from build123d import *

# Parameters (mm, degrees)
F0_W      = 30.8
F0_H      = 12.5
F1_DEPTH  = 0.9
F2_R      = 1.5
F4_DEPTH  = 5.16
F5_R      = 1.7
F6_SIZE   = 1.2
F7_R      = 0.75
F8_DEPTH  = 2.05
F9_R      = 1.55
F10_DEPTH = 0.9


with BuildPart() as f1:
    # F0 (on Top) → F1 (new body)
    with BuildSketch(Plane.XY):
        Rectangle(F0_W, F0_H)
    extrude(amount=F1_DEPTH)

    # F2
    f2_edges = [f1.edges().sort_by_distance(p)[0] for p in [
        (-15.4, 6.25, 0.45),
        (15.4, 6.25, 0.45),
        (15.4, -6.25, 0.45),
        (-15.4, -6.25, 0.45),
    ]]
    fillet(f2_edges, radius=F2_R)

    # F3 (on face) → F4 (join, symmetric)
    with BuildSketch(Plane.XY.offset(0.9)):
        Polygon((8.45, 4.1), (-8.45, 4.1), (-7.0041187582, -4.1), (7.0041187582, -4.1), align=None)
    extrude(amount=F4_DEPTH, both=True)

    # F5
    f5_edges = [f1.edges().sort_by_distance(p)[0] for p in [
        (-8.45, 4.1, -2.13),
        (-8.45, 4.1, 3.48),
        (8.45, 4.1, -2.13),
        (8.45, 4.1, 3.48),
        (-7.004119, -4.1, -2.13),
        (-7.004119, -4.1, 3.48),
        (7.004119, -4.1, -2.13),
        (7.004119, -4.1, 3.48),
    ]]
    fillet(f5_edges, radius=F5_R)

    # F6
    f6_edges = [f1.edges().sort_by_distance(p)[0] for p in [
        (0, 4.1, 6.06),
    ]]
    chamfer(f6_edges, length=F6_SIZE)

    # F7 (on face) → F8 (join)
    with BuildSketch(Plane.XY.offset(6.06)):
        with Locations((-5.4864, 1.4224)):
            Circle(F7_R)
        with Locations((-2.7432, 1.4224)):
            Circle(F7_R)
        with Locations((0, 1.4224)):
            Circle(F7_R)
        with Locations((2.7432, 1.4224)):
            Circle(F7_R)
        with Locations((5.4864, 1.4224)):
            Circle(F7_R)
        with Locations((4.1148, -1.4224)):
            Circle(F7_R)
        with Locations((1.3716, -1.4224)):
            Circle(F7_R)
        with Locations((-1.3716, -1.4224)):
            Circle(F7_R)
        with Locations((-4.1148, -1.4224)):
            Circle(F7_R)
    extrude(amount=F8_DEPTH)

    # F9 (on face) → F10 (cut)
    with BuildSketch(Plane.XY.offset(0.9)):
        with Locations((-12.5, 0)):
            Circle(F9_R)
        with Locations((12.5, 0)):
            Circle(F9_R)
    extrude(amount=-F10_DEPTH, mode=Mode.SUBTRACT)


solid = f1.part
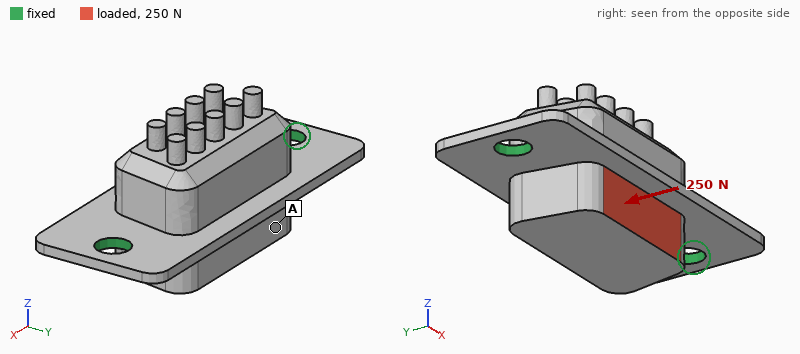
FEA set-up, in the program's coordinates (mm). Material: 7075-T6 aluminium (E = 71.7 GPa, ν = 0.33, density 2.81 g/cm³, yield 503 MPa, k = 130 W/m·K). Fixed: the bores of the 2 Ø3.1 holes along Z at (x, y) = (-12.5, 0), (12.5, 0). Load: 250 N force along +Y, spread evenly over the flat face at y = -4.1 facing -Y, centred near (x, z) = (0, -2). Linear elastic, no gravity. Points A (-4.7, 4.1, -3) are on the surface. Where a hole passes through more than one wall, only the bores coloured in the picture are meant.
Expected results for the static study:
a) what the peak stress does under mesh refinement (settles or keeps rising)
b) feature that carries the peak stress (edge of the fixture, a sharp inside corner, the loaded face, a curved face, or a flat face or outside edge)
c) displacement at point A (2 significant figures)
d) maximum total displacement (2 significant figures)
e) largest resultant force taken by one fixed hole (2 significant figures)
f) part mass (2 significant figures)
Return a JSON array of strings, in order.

["keeps rising", "edge of the fixture", "53 µm", "73 µm", "130 N", "4.2 g"]
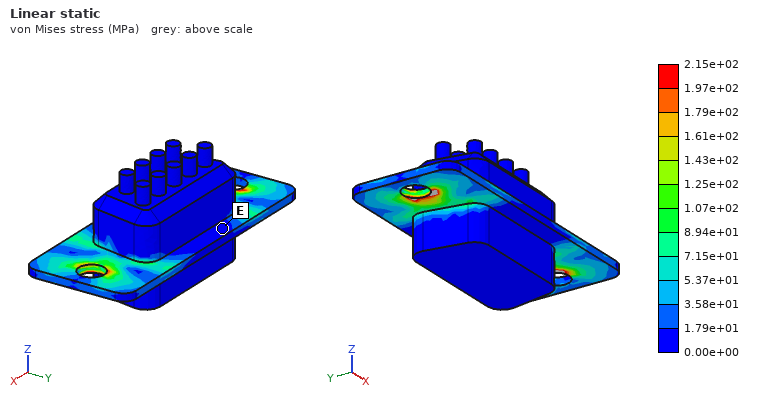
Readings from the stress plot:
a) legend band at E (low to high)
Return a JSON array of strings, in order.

["0.00e+00 to 1.79e+01 MPa"]
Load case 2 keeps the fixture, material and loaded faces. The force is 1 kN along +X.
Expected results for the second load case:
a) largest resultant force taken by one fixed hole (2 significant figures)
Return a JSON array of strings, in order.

["550 N"]
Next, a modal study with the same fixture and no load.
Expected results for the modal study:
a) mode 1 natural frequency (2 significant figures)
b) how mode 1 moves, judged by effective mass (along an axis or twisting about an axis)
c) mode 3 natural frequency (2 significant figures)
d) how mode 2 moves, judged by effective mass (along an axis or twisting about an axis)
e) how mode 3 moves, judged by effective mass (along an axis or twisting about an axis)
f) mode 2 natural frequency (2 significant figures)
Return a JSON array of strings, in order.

["5300 Hz", "twisting about X", "16 kHz", "along Z", "twisting about Y", "8900 Hz"]
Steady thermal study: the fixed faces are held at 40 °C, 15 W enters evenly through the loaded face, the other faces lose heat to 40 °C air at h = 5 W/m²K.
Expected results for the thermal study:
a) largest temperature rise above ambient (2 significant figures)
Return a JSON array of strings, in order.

["40 K"]
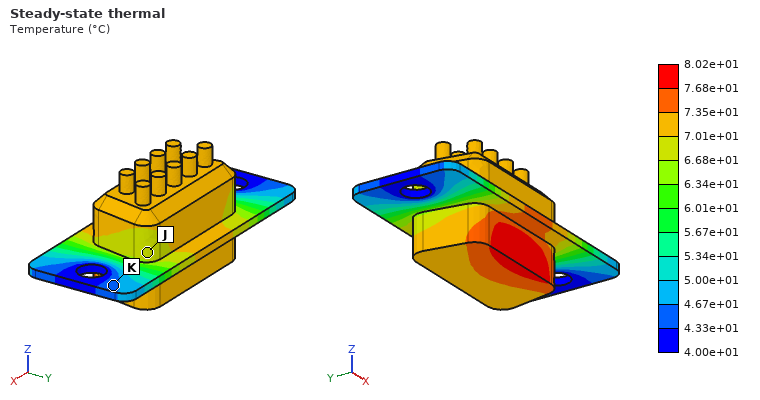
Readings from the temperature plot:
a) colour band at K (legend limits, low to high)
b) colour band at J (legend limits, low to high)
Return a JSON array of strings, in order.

["4.33e+01 to 4.67e+01 °C", "6.68e+01 to 7.01e+01 °C"]
